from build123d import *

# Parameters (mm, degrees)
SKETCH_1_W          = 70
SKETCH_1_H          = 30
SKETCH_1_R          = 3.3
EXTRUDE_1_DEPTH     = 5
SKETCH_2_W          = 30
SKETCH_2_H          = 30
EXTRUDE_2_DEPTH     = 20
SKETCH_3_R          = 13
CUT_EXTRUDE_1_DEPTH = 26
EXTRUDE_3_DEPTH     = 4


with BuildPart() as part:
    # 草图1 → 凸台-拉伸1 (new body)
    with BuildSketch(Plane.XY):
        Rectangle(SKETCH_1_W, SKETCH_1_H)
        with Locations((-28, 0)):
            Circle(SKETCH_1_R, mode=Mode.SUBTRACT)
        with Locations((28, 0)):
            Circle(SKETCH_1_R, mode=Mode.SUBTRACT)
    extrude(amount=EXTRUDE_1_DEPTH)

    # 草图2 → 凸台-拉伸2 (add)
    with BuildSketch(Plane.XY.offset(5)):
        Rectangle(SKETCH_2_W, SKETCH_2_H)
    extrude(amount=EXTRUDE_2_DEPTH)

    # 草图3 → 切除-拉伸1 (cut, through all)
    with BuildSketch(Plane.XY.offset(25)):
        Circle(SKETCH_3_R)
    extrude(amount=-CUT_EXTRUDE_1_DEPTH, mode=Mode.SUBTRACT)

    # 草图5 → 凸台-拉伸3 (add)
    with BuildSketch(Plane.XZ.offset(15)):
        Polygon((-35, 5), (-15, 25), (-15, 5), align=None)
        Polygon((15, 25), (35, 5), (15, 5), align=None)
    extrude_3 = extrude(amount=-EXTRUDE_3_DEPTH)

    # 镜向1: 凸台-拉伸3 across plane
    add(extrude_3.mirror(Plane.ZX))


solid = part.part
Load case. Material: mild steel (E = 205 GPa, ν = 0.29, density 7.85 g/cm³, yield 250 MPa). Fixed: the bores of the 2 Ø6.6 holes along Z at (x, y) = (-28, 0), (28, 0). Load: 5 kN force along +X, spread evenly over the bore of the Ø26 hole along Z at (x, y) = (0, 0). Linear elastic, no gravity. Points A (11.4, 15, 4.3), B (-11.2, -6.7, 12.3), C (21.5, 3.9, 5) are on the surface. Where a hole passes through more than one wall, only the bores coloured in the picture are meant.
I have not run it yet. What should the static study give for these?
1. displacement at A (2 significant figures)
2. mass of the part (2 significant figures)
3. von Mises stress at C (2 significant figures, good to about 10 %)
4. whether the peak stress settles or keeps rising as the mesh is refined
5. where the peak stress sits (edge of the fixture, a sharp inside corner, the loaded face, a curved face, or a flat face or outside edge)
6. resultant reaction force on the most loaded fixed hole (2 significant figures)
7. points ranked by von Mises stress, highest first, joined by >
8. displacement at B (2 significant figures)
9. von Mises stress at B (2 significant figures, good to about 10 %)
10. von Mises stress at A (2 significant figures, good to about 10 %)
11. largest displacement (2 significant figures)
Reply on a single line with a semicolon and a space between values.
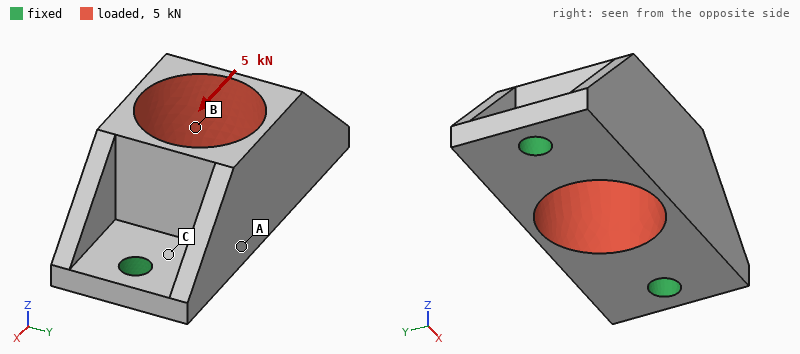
2.7 µm; 140 g; 36 MPa; keeps rising; edge of the fixture; 2.7 kN; C > B > A; 4.8 µm; 25 MPa; 11 MPa; 9.9 µm
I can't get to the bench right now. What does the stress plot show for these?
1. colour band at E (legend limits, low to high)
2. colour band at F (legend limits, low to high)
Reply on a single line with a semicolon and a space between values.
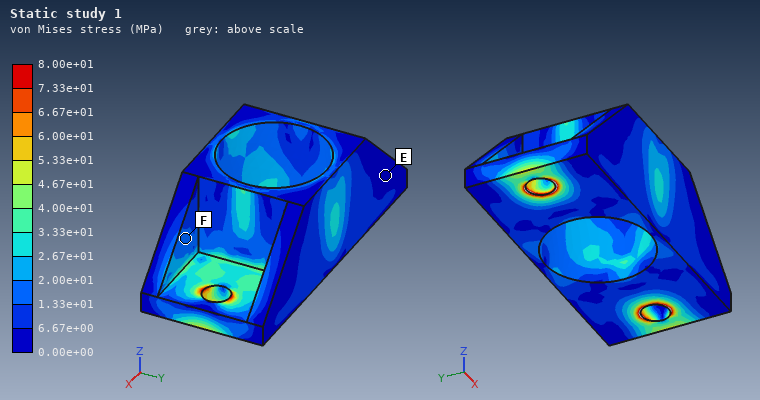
0.00e+00 to 6.67e+00 MPa; 1.33e+01 to 2.00e+01 MPa
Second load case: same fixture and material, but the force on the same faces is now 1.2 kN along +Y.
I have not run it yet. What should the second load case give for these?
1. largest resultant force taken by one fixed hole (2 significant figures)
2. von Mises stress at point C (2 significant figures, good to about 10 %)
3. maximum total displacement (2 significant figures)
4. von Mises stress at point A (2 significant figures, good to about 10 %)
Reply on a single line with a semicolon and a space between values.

600 N; 27 MPa; 15 µm; 9.6 MPa
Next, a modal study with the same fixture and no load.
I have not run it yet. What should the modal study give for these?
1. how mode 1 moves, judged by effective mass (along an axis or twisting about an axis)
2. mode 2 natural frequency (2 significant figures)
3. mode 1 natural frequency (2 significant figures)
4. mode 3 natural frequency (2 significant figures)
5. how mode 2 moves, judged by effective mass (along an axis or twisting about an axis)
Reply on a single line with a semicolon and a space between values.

along Y; 10 kHz; 5100 Hz; 11 kHz; along Z
